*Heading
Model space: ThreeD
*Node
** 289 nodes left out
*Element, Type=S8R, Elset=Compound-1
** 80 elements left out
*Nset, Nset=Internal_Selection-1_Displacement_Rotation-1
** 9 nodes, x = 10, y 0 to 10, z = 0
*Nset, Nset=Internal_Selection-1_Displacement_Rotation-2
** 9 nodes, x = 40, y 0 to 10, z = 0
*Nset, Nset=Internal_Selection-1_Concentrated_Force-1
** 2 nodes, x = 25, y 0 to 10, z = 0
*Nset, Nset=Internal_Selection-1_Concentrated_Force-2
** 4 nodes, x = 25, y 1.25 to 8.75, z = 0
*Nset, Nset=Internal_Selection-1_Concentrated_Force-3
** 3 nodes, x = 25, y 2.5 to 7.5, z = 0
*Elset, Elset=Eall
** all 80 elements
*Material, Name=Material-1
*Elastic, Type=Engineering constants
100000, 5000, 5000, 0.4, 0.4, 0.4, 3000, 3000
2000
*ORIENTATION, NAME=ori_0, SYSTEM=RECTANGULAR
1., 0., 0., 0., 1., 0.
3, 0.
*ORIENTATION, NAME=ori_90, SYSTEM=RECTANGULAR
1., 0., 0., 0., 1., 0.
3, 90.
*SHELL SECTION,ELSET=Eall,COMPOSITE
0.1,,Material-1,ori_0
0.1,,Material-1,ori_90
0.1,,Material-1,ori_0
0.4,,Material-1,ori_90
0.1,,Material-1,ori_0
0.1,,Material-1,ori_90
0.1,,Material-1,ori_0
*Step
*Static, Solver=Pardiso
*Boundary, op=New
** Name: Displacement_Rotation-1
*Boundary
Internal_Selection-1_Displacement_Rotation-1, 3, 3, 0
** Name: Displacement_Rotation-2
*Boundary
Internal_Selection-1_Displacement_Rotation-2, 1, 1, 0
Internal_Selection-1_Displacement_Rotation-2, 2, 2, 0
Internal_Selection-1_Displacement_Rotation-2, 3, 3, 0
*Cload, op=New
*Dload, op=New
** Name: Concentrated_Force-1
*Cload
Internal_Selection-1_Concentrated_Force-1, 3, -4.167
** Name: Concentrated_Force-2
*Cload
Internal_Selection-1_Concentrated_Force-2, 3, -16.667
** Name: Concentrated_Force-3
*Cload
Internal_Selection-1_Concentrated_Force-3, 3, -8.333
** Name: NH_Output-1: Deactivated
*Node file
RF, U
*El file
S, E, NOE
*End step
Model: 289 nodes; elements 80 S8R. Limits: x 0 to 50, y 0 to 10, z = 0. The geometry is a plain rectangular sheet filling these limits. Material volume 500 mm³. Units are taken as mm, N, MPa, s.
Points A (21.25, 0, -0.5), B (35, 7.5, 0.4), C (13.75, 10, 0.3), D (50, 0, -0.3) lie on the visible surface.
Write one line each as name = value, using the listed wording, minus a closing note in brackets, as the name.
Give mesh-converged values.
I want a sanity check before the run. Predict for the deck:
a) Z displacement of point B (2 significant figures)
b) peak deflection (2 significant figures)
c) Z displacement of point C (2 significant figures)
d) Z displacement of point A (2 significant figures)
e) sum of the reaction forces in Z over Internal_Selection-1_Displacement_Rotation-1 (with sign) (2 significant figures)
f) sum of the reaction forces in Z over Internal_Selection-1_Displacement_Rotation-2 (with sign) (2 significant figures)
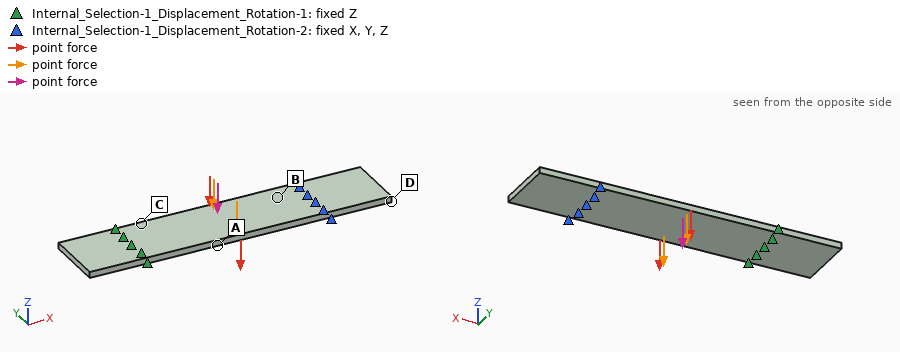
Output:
Z displacement of point B = -0.50 mm
peak deflection = 1.1 mm
Z displacement of point C = -0.38 mm
Z displacement of point A = -0.96 mm
sum of the reaction forces in Z over Internal_Selection-1_Displacement_Rotation-1 (with sign) = 50 N
sum of the reaction forces in Z over Internal_Selection-1_Displacement_Rotation-2 (with sign) = 50 N
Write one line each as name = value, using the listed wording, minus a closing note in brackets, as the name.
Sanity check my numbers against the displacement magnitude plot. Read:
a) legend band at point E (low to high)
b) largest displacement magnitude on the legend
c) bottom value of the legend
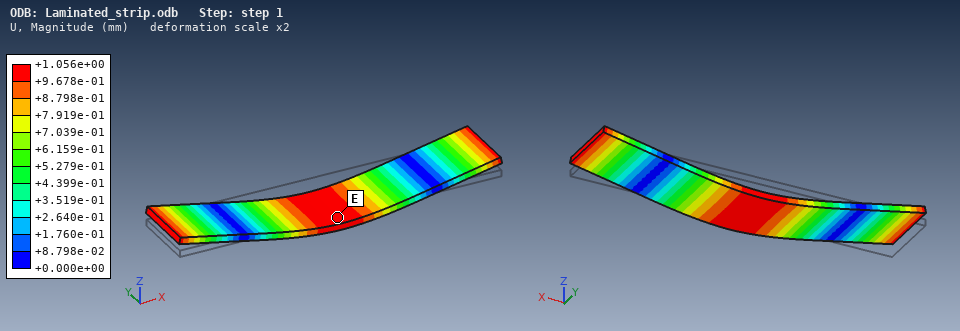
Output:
legend band at point E = +9.678e-01 to +1.056e+00 mm
largest displacement magnitude on the legend = +1.056e+00 mm
bottom value of the legend = +0.000e+00 mm
